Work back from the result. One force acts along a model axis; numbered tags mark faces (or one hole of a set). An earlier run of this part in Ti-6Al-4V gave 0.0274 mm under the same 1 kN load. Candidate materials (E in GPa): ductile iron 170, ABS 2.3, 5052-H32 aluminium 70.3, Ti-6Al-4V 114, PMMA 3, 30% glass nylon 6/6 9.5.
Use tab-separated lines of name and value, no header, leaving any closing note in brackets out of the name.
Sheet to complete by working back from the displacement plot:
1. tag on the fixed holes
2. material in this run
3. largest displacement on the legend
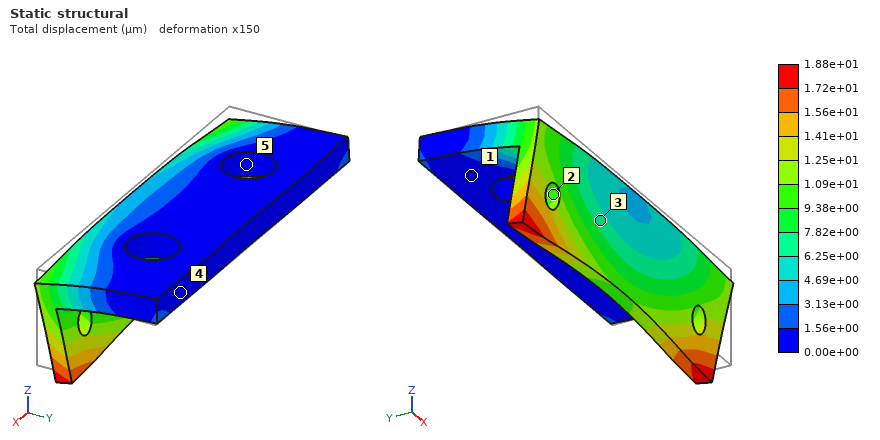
tag on the fixed holes	5
material in this run	ductile iron
largest displacement on the legend	1.88e+01 µm
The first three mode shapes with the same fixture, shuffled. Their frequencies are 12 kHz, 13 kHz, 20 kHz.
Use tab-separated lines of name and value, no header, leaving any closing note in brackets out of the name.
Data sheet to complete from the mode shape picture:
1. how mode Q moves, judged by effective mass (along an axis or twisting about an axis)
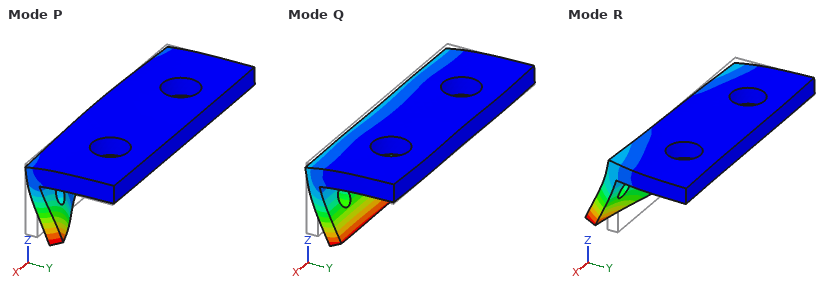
how mode Q moves, judged by effective mass	along Y
